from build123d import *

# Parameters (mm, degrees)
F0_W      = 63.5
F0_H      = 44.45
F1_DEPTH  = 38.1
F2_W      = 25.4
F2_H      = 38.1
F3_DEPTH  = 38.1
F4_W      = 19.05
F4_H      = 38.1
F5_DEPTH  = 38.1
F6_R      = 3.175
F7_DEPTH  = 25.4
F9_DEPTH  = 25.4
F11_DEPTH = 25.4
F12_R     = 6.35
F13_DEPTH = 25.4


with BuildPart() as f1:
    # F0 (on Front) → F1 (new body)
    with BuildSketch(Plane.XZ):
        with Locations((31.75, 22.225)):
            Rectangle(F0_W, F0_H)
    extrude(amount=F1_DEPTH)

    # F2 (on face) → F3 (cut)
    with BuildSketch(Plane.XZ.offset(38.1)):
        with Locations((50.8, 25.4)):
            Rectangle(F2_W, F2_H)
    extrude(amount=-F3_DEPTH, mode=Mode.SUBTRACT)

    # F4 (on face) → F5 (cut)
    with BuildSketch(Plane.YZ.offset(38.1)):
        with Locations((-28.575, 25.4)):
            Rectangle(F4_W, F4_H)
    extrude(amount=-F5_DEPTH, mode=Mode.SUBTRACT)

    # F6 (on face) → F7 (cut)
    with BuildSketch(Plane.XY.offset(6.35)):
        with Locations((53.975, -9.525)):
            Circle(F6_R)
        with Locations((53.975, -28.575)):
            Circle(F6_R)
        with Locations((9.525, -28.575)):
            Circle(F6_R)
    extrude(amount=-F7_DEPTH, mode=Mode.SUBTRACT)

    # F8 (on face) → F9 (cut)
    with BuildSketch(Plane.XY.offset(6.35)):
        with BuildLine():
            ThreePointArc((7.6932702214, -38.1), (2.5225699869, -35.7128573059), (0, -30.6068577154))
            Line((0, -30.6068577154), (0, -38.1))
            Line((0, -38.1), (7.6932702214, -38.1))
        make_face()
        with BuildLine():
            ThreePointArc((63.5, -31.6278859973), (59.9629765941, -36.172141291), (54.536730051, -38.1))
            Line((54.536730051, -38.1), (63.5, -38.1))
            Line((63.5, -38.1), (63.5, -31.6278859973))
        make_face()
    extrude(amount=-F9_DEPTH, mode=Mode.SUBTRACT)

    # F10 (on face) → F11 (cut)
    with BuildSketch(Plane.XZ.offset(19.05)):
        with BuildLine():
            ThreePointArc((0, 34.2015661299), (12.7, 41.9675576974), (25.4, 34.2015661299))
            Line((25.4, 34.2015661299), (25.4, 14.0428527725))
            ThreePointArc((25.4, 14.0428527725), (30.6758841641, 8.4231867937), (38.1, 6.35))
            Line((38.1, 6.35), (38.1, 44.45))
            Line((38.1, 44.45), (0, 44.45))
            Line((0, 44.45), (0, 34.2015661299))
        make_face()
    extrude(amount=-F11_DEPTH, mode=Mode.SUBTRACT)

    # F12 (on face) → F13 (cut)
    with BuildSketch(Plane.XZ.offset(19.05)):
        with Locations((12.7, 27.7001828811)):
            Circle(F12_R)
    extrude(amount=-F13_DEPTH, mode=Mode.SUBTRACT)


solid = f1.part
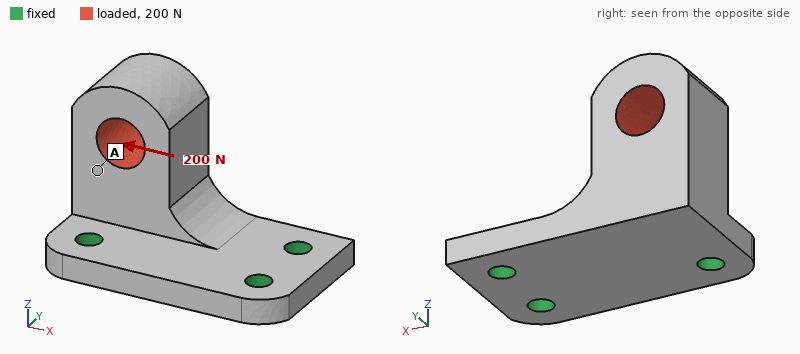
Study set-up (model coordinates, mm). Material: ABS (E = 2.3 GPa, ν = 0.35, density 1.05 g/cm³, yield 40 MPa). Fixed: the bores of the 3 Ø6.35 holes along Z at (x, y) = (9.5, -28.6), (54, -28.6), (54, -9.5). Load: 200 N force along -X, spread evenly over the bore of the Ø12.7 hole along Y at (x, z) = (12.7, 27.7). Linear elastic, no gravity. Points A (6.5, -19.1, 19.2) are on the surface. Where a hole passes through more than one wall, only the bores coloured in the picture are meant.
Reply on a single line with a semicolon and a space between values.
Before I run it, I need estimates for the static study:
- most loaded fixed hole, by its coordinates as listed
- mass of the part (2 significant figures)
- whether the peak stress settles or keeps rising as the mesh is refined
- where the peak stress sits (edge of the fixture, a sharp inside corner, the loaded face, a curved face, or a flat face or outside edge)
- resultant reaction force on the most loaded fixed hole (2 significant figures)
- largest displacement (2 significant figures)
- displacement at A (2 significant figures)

(9.5, -28.6); 30 g; keeps rising; edge of the fixture; 130 N; 0.34 mm; 0.14 mm
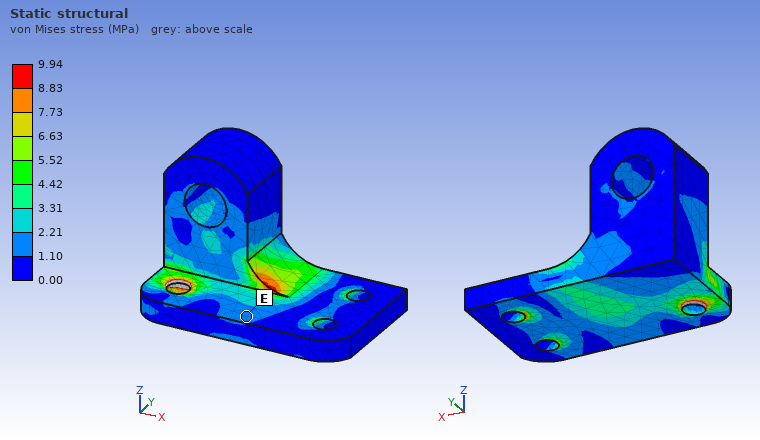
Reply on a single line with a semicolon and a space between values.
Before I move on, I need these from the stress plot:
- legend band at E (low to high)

1.10 to 2.21 MPa
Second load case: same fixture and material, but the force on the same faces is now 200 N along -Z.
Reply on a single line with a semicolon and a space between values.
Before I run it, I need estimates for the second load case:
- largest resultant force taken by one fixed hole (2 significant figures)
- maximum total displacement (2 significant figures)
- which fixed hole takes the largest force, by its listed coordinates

160 N; 0.47 mm; (9.5, -28.6)
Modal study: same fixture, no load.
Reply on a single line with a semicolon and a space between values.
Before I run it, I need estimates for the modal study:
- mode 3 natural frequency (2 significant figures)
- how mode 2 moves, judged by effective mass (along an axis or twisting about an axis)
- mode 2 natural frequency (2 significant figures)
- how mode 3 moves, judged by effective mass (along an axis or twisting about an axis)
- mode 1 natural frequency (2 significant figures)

2800 Hz; along X; 1600 Hz; along Z; 750 Hz
